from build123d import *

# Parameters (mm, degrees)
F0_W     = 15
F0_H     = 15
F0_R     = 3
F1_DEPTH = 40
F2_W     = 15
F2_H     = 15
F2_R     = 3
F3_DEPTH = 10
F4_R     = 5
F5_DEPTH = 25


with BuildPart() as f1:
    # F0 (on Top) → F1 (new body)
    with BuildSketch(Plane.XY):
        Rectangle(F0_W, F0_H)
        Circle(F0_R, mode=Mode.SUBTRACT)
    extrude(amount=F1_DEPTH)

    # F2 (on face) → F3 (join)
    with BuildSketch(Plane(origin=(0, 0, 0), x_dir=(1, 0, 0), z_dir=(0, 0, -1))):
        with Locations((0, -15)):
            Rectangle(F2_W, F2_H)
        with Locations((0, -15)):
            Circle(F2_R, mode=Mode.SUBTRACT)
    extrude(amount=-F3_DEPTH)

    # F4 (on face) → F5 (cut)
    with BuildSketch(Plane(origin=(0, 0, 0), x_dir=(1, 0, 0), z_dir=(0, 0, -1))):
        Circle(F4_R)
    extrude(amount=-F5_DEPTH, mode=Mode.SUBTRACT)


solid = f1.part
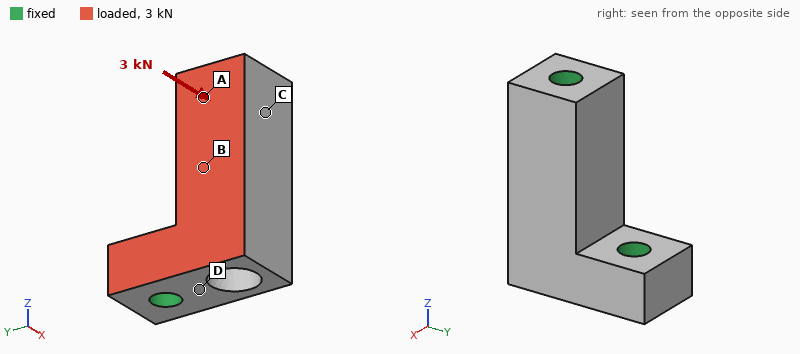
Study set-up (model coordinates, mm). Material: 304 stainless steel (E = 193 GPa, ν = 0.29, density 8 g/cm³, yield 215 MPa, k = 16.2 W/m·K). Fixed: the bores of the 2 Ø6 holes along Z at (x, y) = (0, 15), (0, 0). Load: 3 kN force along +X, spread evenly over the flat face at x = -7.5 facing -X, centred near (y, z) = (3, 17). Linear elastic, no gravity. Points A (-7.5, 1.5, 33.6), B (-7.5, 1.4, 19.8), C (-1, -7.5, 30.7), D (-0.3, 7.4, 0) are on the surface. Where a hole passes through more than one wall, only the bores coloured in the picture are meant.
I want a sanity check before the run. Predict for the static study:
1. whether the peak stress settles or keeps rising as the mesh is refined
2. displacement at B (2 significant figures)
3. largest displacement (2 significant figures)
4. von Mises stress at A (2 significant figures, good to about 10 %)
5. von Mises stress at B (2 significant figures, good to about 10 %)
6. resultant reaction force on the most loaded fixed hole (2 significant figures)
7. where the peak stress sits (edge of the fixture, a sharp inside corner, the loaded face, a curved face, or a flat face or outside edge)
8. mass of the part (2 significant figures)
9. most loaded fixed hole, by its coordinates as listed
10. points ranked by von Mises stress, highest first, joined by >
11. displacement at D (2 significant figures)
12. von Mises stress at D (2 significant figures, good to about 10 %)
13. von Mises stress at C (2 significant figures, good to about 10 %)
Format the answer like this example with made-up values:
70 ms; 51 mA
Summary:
keeps rising; 2.2 µm; 5.7 µm; 7.6 MPa; 16 MPa; 1.7 kN; edge of the fixture; 69 g; (0, 0); D > B > A > C; 1.1 µm; 22 MPa; 4.9 MPa
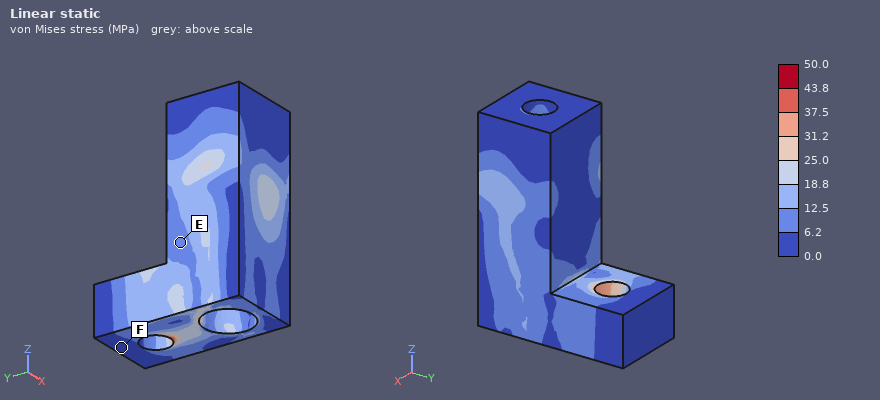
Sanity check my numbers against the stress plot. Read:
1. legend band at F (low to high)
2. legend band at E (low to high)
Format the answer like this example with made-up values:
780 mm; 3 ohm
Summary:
0.0 to 6.2 MPa; 6.2 to 12.5 MPa
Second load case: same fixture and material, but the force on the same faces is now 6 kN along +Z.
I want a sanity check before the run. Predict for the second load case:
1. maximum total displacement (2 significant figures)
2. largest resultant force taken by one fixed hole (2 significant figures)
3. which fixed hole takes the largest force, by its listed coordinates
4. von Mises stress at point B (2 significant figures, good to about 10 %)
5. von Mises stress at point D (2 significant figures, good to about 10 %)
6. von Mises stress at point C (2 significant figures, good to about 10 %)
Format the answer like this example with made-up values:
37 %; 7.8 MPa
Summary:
8.1 µm; 4.2 kN; (0, 0); 34 MPa; 33 MPa; 12 MPa
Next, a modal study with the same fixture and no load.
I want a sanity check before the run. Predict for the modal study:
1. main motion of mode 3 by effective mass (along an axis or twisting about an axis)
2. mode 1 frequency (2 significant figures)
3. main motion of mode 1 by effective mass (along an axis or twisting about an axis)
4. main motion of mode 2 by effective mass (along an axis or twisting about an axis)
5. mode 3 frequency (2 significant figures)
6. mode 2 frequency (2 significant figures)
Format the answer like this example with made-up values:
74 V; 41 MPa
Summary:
along Z; 19 kHz; along X; along Y; 41 kHz; 37 kHz
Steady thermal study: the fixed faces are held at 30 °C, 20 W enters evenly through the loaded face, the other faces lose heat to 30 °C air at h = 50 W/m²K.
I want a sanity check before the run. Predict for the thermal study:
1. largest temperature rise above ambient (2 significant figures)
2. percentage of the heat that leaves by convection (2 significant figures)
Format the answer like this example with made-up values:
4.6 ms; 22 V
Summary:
41 K; 11 %
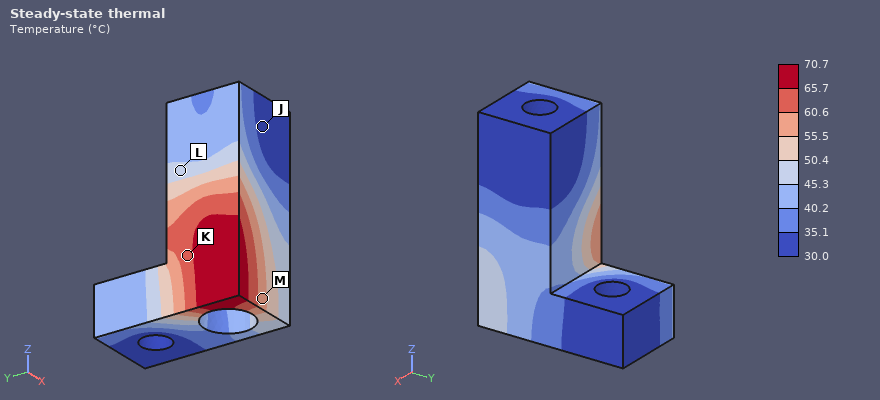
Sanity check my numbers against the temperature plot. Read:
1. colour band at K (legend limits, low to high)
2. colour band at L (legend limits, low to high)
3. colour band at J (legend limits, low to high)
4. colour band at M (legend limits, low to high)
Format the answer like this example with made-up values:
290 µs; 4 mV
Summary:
60.6 to 65.7 °C; 45.3 to 50.4 °C; 30.0 to 35.1 °C; 55.5 to 60.6 °C
